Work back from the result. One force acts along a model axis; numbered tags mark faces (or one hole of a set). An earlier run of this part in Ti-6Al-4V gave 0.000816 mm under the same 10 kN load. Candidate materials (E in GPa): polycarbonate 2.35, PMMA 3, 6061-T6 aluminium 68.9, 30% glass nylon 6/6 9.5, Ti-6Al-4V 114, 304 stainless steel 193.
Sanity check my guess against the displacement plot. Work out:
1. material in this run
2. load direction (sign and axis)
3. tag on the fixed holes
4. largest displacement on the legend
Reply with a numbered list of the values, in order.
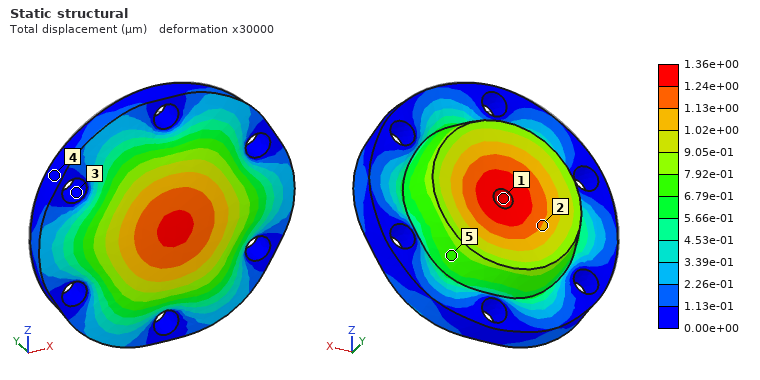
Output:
1. 6061-T6 aluminium
2. -Y
3. 3
4. 1.36e+00 µm
